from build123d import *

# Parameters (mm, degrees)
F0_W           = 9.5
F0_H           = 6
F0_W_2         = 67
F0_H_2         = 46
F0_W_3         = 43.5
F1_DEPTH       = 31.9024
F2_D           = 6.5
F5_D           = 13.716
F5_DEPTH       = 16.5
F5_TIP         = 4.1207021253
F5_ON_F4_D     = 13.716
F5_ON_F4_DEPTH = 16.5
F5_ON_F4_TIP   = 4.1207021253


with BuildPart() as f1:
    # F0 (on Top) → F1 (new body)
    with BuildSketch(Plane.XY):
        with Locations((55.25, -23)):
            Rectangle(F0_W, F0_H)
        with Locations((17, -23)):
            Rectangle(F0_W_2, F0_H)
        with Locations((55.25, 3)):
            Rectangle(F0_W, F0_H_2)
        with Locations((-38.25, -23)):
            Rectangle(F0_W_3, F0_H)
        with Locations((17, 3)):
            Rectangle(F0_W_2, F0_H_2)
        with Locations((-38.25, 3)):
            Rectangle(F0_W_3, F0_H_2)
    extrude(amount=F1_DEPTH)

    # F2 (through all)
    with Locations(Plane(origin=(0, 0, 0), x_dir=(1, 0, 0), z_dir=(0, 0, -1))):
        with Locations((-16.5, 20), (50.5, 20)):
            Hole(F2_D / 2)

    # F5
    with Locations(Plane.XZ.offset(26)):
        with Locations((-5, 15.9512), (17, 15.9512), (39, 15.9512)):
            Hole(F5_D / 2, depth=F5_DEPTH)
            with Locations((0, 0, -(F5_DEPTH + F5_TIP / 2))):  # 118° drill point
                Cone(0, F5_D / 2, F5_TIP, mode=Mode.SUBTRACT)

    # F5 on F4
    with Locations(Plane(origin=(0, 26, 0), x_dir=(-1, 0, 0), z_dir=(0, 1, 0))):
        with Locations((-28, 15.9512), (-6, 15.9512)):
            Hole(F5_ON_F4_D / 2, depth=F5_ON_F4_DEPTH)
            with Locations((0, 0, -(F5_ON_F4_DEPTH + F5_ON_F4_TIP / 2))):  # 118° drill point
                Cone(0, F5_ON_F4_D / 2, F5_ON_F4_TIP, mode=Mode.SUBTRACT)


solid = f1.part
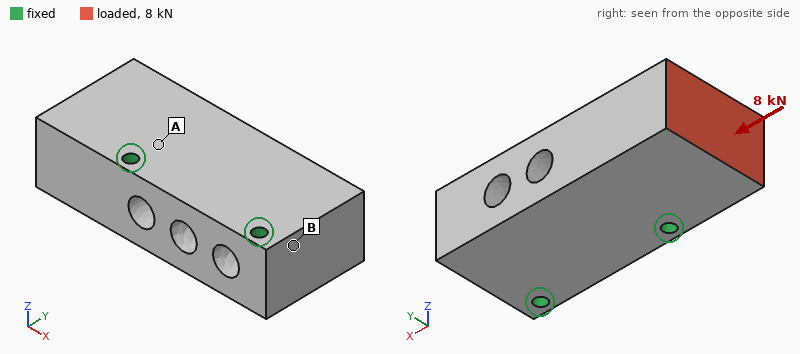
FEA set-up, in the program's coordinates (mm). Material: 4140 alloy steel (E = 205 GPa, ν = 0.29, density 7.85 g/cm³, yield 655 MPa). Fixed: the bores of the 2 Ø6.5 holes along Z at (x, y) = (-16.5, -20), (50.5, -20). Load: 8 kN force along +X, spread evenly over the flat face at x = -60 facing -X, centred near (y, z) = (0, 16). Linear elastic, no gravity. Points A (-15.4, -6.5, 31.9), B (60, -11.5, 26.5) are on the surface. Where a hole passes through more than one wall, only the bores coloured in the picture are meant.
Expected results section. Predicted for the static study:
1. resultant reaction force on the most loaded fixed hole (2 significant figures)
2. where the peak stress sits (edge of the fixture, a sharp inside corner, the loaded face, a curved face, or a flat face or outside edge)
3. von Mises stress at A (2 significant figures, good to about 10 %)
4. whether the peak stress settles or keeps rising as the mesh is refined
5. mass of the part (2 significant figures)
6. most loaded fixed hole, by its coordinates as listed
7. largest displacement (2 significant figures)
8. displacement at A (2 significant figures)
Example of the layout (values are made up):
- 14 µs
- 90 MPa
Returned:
- 5.8 kN
- edge of the fixture
- 5.2 MPa
- keeps rising
- 1.4 kg
- (-16.5, -20)
- 4.7 µm
- 1.0 µm
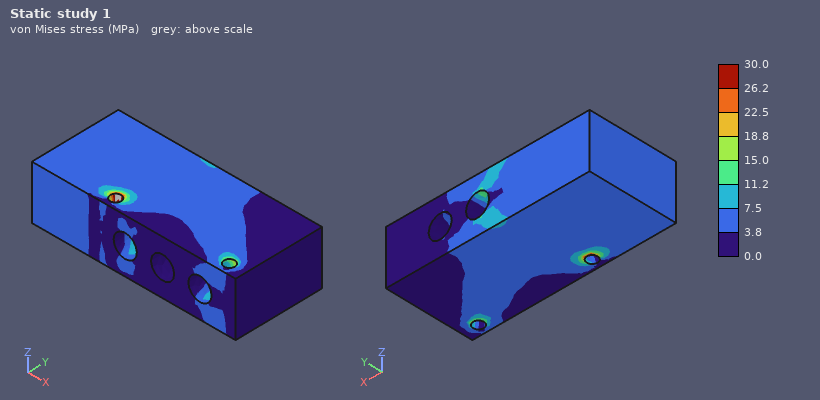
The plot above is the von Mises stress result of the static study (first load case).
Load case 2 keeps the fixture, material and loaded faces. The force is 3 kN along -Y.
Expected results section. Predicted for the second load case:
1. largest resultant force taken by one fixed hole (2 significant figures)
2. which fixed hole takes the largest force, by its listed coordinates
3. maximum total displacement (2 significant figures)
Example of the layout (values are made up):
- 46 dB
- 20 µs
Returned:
- 5.0 kN
- (-16.5, -20)
- 5.8 µm
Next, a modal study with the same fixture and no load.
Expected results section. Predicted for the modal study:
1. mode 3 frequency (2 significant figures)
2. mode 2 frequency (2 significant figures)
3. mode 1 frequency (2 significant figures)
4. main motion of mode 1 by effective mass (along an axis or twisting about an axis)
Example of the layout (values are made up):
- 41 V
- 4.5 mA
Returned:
- 7700 Hz
- 7200 Hz
- 5600 Hz
- along Z
